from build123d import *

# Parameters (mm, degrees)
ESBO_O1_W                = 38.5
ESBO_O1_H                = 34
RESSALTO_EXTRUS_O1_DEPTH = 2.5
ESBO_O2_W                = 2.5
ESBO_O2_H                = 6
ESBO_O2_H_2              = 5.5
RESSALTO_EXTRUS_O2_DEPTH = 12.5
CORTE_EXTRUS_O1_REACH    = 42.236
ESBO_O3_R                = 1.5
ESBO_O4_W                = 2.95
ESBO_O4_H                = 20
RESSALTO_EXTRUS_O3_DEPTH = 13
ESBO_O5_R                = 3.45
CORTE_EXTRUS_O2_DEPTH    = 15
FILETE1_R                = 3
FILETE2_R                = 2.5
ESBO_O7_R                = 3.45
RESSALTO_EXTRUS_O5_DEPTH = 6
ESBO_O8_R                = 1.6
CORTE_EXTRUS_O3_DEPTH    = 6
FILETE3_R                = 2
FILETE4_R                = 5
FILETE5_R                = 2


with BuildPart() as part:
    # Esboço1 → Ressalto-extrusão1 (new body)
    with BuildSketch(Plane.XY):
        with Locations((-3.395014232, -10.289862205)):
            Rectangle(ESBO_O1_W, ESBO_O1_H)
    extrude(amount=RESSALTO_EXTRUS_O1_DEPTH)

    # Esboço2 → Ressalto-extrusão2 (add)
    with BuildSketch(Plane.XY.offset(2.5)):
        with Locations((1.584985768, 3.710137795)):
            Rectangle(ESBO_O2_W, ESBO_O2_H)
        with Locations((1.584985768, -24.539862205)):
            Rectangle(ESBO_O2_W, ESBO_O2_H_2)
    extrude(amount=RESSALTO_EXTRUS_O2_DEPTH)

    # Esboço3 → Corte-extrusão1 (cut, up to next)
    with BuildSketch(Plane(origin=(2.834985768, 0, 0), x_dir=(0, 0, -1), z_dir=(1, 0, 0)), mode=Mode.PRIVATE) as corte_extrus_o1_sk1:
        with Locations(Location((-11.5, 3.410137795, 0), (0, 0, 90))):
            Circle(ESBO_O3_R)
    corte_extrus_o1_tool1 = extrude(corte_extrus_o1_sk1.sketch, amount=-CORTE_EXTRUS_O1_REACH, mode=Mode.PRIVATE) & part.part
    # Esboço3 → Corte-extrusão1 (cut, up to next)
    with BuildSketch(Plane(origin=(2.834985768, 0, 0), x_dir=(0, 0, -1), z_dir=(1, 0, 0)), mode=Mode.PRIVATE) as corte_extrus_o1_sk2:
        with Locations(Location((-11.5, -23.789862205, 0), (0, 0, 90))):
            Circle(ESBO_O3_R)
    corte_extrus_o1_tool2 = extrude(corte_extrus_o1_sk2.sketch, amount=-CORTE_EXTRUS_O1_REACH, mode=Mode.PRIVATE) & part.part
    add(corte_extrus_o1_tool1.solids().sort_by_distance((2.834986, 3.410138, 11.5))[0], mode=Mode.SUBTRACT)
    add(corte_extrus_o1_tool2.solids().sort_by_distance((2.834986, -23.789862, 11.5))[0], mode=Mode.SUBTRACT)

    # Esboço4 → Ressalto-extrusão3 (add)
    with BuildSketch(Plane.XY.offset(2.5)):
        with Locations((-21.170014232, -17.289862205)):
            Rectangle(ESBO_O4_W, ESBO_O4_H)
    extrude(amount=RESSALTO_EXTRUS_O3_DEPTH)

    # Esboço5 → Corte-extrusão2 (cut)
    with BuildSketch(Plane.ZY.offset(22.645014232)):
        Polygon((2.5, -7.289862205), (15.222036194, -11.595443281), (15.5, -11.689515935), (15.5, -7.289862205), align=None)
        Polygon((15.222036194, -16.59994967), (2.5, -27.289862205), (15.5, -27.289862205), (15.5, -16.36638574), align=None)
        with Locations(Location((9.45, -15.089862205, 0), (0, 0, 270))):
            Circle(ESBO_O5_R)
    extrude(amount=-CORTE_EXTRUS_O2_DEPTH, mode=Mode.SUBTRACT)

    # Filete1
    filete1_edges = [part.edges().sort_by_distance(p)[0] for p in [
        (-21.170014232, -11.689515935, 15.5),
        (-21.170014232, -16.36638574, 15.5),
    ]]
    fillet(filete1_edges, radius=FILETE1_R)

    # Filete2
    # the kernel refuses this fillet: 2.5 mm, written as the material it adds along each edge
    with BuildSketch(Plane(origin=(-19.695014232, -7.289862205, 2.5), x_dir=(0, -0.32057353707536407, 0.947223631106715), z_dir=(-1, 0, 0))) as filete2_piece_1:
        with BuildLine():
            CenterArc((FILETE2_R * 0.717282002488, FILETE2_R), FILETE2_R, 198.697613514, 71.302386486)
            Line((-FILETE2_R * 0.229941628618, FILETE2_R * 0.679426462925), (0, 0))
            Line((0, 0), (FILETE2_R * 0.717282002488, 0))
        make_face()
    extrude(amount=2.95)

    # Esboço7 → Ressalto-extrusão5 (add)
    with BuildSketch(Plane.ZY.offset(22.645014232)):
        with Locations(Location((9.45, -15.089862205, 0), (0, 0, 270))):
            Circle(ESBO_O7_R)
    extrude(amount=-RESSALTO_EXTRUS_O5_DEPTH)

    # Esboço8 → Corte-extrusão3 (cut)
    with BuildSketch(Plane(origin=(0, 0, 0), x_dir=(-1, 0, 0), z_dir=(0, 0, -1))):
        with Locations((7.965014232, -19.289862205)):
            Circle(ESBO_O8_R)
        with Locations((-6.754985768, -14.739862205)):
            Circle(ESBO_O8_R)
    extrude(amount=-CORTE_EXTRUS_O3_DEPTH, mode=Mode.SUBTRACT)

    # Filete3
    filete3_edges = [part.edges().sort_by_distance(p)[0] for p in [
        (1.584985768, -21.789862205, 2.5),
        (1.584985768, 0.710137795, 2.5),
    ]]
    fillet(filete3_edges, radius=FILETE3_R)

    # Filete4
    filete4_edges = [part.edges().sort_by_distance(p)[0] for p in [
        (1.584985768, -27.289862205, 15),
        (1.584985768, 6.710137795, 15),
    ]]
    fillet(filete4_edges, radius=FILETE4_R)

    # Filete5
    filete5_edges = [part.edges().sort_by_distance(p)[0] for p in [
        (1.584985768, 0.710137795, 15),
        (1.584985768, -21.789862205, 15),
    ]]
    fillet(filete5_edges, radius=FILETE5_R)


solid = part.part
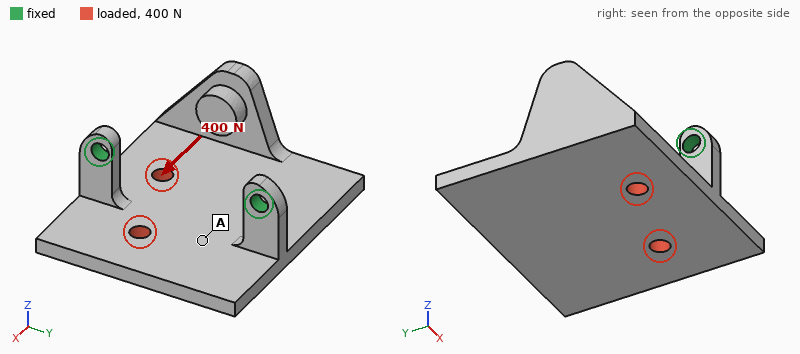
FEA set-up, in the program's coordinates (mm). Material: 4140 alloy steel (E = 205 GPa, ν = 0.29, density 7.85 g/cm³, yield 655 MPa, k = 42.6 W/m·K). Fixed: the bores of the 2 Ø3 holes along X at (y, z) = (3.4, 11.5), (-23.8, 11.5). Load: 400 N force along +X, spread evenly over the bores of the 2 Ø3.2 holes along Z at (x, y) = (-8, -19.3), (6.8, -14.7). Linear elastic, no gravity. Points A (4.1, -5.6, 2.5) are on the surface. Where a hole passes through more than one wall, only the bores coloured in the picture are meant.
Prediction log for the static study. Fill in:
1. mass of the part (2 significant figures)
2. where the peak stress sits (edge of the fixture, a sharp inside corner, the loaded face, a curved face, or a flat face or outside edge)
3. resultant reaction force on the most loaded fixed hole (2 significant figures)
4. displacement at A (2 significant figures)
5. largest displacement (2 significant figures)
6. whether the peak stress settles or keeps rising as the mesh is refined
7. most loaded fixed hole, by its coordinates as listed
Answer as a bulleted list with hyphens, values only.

- 32 g
- edge of the fixture
- 290 N
- 0.031 mm
- 0.15 mm
- keeps rising
- (-23.8, 11.5)
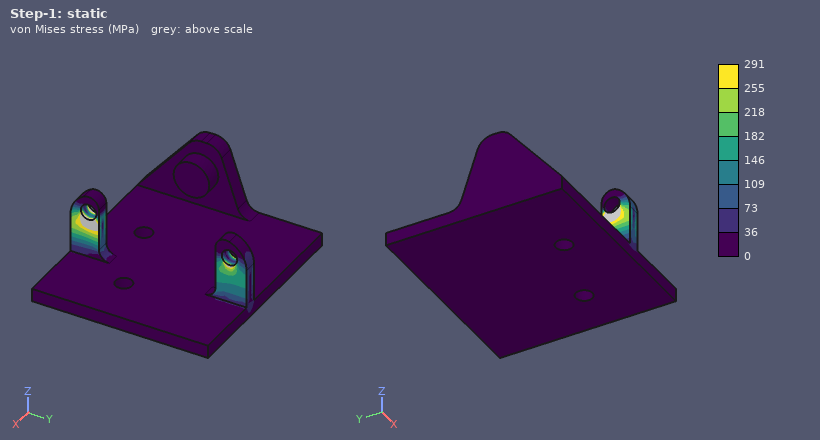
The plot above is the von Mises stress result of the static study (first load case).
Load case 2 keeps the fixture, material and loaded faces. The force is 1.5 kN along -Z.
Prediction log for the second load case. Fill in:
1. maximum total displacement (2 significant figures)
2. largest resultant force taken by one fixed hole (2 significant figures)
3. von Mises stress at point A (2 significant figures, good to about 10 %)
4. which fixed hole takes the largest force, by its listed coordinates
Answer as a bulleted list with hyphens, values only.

- 0.36 mm
- 1.2 kN
- 52 MPa
- (-23.8, 11.5)
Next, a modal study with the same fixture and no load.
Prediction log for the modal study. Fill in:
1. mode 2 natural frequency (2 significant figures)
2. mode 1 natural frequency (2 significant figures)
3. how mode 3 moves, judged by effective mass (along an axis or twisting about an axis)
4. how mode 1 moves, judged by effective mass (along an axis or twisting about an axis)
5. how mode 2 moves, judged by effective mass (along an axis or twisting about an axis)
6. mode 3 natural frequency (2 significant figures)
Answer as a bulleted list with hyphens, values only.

- 3200 Hz
- 1000 Hz
- along X
- along Z
- along Y
- 4000 Hz
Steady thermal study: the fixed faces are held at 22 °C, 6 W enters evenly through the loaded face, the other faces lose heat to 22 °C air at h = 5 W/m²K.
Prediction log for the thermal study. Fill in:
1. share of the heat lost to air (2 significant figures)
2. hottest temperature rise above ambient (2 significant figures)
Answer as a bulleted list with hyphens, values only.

- 13 %
- 57 K
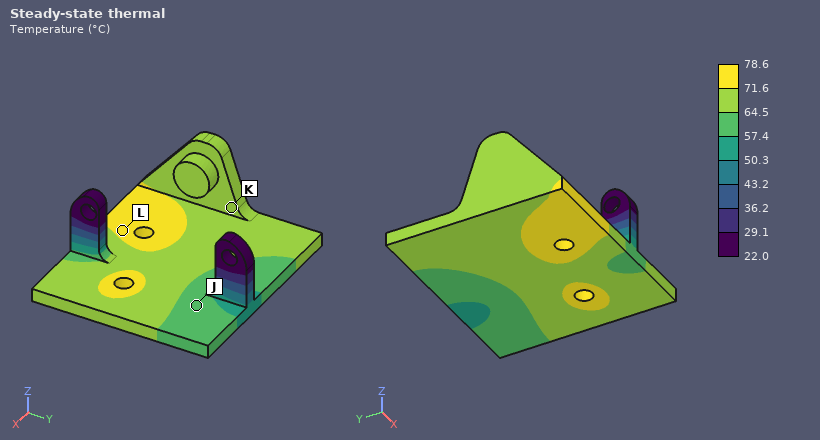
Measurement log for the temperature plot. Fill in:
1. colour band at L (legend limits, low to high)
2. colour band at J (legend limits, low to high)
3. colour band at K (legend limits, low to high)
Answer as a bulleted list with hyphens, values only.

- 71.6 to 78.6 °C
- 57.4 to 64.5 °C
- 64.5 to 71.6 °C
